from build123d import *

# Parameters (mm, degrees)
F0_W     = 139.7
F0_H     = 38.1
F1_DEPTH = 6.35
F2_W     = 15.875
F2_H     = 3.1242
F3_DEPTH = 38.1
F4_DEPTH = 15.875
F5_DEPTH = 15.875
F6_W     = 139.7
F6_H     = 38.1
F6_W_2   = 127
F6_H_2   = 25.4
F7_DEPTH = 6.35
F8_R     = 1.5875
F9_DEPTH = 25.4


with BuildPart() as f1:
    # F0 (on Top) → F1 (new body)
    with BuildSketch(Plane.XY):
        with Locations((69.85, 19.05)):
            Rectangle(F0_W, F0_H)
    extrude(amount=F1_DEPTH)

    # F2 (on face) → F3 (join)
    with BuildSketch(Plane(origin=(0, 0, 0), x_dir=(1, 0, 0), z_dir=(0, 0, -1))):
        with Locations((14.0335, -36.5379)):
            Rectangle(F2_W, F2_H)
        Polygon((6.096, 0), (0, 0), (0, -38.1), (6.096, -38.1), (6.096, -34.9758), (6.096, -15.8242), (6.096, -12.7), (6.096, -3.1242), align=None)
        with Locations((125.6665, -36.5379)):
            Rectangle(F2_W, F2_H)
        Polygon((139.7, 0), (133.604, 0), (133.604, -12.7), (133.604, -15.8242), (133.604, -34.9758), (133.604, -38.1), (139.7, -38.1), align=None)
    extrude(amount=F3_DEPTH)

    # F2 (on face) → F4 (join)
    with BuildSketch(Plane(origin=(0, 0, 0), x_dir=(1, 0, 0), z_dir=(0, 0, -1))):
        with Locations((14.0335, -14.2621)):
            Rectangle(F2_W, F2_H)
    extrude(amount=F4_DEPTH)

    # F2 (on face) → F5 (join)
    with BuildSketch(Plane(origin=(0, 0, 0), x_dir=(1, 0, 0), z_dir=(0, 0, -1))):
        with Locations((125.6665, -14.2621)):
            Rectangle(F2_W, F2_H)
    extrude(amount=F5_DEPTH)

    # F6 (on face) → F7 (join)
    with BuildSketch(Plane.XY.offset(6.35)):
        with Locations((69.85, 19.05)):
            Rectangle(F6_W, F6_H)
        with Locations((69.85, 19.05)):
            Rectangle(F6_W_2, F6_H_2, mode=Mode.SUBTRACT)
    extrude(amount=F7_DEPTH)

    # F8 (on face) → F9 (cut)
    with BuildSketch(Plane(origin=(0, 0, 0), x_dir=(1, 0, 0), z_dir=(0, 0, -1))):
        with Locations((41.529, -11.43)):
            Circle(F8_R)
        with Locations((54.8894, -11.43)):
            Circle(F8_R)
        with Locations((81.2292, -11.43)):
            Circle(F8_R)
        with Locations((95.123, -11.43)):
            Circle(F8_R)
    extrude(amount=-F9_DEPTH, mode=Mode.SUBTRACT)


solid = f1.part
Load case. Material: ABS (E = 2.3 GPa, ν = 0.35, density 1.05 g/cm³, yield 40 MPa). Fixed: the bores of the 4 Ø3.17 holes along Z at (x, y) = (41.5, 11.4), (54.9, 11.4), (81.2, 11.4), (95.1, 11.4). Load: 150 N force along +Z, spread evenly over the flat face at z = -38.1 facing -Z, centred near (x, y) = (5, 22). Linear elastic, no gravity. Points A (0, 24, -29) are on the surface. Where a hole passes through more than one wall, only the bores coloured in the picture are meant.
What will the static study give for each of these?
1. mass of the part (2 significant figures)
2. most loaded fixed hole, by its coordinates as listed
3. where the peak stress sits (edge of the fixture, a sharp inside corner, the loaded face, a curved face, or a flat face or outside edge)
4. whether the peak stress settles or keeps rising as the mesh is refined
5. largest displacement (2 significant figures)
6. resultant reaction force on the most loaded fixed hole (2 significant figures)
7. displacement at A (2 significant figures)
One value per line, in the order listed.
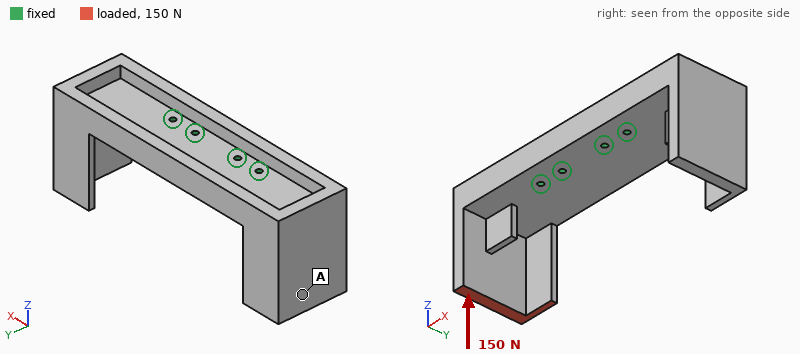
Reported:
73 g
(41.5, 11.4)
edge of the fixture
keeps rising
1.5 mm
320 N
1.2 mm
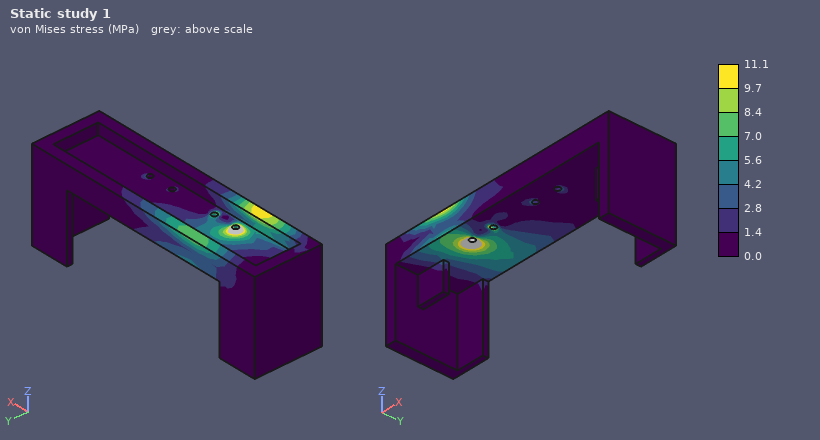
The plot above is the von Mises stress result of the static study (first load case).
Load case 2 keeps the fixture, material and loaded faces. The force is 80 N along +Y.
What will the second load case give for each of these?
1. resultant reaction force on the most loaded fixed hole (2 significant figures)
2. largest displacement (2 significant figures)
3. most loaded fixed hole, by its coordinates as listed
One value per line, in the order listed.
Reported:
120 N
1.7 mm
(41.5, 11.4)
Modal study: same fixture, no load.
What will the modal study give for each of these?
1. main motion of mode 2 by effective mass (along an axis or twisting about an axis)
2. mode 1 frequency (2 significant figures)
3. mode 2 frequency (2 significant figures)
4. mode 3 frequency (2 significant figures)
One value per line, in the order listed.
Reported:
along Z
390 Hz
420 Hz
540 Hz
